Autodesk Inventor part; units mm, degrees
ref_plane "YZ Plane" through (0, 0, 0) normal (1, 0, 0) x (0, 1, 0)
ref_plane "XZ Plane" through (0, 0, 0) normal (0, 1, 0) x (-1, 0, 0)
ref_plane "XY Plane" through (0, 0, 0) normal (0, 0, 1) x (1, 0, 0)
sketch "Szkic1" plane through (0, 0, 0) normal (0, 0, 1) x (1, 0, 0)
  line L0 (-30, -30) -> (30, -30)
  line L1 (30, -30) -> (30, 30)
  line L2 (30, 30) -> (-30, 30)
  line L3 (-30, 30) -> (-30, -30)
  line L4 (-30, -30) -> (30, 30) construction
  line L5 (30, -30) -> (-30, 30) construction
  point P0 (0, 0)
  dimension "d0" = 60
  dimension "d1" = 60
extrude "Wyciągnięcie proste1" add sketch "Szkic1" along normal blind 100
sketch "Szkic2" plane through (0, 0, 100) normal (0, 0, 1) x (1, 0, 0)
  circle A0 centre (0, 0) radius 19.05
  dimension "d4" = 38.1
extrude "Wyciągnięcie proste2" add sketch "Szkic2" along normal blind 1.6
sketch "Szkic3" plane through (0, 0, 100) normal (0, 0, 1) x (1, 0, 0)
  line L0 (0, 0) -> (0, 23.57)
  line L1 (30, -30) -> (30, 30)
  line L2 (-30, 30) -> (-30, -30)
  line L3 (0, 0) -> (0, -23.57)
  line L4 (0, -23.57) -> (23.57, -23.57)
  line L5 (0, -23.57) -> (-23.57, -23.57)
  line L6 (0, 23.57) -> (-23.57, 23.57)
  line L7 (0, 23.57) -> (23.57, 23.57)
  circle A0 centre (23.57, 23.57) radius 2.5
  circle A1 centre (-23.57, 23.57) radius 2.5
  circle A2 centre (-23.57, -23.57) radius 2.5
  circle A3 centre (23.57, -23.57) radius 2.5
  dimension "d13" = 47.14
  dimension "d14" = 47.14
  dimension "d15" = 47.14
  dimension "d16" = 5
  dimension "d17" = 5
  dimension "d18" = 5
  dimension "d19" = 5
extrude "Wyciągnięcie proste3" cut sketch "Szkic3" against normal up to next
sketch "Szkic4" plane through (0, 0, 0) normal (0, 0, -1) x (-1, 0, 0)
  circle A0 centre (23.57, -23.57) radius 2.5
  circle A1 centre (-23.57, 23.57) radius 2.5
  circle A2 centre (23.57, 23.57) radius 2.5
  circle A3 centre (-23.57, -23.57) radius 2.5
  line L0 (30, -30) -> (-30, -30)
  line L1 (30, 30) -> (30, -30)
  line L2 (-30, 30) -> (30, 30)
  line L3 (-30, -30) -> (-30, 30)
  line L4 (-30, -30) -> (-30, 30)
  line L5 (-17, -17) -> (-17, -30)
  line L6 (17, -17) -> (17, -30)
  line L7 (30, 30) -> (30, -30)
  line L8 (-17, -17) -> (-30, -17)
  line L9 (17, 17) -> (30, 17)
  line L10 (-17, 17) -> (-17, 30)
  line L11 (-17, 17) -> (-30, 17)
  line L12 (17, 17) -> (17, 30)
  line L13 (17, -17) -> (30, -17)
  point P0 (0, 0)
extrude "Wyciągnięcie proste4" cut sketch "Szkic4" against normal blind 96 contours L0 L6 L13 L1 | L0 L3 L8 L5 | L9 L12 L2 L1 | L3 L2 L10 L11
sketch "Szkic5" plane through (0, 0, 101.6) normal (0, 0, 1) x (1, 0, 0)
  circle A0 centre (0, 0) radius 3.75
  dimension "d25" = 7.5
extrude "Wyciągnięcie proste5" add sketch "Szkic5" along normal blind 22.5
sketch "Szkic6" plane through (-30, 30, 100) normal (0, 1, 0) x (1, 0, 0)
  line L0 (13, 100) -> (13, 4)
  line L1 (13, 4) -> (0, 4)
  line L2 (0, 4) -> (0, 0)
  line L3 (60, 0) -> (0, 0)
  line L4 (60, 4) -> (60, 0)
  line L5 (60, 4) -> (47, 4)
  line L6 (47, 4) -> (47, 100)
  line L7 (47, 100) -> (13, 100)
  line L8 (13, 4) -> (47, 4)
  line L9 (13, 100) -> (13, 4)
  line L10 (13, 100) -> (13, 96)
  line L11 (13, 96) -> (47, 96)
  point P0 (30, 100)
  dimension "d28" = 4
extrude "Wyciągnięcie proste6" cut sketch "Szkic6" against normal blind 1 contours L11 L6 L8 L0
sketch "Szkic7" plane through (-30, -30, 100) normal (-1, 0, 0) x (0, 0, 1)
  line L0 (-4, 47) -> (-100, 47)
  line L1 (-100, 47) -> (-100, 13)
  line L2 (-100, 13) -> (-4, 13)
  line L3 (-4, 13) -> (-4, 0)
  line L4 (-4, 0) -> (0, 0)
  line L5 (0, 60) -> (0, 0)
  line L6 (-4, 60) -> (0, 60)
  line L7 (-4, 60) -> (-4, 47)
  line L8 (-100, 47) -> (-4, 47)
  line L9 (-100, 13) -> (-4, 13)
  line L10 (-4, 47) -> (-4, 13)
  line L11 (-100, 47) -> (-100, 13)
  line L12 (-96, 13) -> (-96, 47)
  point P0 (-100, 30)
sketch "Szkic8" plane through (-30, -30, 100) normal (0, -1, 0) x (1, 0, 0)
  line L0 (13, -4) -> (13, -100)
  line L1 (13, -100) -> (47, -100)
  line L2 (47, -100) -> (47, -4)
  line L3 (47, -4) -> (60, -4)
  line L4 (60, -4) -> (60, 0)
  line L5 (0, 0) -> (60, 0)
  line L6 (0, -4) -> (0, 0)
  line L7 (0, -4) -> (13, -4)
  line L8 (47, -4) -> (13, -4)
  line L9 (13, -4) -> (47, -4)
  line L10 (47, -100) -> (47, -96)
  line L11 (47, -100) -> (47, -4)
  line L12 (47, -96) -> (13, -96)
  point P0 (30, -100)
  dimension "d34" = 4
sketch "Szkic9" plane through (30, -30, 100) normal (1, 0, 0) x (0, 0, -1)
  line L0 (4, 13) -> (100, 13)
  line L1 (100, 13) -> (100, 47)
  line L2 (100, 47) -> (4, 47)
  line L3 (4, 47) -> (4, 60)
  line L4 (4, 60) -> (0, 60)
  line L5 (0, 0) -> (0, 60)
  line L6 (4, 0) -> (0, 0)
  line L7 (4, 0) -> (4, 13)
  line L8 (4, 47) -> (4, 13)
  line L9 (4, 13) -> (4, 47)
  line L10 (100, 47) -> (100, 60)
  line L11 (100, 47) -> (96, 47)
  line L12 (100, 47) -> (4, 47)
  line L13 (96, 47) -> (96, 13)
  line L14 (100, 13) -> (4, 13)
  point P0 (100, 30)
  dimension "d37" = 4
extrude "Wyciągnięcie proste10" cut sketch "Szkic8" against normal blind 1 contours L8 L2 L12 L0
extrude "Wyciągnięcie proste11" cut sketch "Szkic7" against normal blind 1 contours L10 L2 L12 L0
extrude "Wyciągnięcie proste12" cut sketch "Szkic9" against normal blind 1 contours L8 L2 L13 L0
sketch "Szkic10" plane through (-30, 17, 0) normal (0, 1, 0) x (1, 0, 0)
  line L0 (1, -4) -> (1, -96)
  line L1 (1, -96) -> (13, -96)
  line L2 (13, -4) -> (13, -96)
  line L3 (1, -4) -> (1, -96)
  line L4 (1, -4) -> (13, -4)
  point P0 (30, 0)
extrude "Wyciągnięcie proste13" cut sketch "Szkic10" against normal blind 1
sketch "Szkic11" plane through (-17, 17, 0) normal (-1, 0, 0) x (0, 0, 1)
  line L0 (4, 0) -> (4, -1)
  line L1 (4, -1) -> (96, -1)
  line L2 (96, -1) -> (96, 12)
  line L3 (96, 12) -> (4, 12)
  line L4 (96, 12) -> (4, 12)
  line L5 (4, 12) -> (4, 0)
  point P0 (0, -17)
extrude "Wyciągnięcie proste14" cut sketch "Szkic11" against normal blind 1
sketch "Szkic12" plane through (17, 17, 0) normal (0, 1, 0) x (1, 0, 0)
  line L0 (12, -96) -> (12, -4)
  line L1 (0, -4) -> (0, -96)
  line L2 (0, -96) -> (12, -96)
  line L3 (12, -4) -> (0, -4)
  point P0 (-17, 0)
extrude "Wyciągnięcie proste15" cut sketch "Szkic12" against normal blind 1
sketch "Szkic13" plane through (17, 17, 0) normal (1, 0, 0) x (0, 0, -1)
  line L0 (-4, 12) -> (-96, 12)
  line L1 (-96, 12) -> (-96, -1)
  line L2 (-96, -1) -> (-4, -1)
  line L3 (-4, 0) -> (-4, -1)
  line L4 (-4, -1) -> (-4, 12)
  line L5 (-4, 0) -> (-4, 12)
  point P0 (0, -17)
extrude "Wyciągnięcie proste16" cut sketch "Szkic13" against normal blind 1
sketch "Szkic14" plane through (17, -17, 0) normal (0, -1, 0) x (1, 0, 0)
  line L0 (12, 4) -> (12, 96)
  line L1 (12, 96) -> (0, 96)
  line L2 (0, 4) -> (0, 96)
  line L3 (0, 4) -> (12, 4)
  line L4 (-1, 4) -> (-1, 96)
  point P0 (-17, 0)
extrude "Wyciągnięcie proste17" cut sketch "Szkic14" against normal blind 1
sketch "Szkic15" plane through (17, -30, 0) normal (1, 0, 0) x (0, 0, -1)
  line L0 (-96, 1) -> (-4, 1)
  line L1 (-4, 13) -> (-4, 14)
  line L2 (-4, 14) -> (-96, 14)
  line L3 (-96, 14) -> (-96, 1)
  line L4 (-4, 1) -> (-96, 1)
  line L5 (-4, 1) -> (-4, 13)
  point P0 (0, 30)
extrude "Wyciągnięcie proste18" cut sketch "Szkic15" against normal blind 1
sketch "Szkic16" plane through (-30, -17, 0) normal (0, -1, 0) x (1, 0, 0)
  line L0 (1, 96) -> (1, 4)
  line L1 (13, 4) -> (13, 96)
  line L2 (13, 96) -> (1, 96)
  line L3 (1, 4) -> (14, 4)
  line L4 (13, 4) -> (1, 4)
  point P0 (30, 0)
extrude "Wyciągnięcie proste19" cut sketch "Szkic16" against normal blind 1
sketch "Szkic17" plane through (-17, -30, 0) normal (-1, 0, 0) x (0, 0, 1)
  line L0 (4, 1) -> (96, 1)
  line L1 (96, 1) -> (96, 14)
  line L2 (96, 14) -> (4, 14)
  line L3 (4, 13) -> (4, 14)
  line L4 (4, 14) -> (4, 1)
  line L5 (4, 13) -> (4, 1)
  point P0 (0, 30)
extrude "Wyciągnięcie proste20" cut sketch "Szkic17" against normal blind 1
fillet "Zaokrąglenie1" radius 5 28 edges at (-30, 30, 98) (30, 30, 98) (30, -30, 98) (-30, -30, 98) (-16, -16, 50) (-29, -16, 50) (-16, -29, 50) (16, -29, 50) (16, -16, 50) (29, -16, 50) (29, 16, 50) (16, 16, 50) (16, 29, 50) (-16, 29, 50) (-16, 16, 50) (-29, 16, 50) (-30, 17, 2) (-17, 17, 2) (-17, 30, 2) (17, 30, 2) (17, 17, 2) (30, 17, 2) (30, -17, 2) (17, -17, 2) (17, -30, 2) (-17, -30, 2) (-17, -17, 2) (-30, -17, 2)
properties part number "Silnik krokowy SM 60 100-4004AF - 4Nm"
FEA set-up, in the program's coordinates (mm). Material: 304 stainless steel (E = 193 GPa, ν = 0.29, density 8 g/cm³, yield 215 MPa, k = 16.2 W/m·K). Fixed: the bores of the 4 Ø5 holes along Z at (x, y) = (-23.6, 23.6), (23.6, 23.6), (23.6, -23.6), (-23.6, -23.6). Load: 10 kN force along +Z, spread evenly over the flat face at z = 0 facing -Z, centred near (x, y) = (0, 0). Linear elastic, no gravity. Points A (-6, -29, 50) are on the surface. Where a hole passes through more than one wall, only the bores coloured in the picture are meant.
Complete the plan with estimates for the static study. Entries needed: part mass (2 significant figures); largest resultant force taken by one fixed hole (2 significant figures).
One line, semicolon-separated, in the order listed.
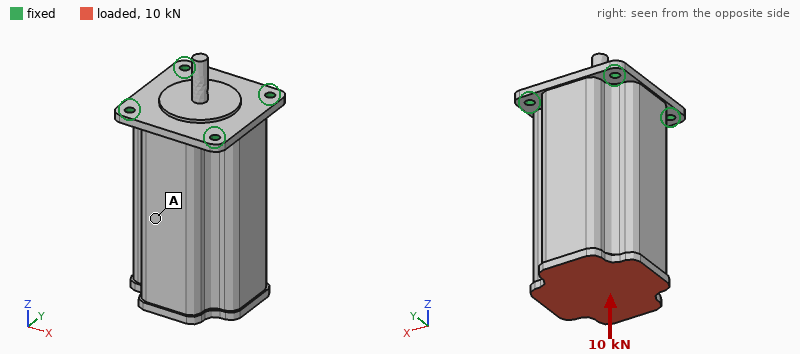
2.2 kg; 2.7 kN
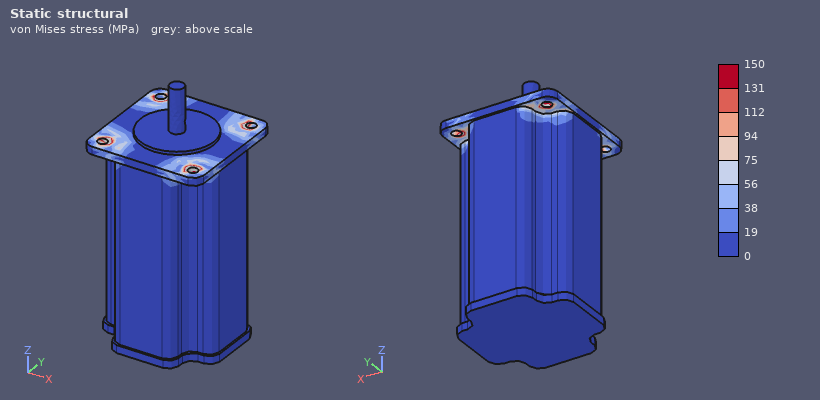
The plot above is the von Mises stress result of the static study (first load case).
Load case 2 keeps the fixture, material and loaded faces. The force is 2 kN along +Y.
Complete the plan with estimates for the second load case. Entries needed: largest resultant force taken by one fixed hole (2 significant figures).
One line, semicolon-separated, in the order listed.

2.4 kN
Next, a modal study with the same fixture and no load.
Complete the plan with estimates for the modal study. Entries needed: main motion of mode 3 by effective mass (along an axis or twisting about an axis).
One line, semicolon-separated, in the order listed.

along Z
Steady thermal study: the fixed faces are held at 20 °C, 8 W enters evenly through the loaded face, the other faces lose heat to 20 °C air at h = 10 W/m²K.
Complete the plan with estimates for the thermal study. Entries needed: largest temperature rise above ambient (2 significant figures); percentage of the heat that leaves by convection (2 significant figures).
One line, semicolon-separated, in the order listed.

22 K; 42 %
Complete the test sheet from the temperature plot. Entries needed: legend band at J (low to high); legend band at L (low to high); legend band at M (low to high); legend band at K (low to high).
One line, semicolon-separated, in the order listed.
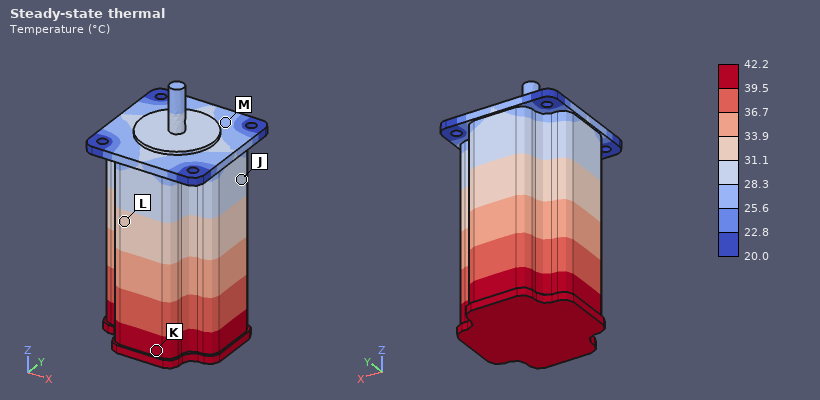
28.3 to 31.1 °C; 31.1 to 33.9 °C; 25.6 to 28.3 °C; 39.5 to 42.2 °C
